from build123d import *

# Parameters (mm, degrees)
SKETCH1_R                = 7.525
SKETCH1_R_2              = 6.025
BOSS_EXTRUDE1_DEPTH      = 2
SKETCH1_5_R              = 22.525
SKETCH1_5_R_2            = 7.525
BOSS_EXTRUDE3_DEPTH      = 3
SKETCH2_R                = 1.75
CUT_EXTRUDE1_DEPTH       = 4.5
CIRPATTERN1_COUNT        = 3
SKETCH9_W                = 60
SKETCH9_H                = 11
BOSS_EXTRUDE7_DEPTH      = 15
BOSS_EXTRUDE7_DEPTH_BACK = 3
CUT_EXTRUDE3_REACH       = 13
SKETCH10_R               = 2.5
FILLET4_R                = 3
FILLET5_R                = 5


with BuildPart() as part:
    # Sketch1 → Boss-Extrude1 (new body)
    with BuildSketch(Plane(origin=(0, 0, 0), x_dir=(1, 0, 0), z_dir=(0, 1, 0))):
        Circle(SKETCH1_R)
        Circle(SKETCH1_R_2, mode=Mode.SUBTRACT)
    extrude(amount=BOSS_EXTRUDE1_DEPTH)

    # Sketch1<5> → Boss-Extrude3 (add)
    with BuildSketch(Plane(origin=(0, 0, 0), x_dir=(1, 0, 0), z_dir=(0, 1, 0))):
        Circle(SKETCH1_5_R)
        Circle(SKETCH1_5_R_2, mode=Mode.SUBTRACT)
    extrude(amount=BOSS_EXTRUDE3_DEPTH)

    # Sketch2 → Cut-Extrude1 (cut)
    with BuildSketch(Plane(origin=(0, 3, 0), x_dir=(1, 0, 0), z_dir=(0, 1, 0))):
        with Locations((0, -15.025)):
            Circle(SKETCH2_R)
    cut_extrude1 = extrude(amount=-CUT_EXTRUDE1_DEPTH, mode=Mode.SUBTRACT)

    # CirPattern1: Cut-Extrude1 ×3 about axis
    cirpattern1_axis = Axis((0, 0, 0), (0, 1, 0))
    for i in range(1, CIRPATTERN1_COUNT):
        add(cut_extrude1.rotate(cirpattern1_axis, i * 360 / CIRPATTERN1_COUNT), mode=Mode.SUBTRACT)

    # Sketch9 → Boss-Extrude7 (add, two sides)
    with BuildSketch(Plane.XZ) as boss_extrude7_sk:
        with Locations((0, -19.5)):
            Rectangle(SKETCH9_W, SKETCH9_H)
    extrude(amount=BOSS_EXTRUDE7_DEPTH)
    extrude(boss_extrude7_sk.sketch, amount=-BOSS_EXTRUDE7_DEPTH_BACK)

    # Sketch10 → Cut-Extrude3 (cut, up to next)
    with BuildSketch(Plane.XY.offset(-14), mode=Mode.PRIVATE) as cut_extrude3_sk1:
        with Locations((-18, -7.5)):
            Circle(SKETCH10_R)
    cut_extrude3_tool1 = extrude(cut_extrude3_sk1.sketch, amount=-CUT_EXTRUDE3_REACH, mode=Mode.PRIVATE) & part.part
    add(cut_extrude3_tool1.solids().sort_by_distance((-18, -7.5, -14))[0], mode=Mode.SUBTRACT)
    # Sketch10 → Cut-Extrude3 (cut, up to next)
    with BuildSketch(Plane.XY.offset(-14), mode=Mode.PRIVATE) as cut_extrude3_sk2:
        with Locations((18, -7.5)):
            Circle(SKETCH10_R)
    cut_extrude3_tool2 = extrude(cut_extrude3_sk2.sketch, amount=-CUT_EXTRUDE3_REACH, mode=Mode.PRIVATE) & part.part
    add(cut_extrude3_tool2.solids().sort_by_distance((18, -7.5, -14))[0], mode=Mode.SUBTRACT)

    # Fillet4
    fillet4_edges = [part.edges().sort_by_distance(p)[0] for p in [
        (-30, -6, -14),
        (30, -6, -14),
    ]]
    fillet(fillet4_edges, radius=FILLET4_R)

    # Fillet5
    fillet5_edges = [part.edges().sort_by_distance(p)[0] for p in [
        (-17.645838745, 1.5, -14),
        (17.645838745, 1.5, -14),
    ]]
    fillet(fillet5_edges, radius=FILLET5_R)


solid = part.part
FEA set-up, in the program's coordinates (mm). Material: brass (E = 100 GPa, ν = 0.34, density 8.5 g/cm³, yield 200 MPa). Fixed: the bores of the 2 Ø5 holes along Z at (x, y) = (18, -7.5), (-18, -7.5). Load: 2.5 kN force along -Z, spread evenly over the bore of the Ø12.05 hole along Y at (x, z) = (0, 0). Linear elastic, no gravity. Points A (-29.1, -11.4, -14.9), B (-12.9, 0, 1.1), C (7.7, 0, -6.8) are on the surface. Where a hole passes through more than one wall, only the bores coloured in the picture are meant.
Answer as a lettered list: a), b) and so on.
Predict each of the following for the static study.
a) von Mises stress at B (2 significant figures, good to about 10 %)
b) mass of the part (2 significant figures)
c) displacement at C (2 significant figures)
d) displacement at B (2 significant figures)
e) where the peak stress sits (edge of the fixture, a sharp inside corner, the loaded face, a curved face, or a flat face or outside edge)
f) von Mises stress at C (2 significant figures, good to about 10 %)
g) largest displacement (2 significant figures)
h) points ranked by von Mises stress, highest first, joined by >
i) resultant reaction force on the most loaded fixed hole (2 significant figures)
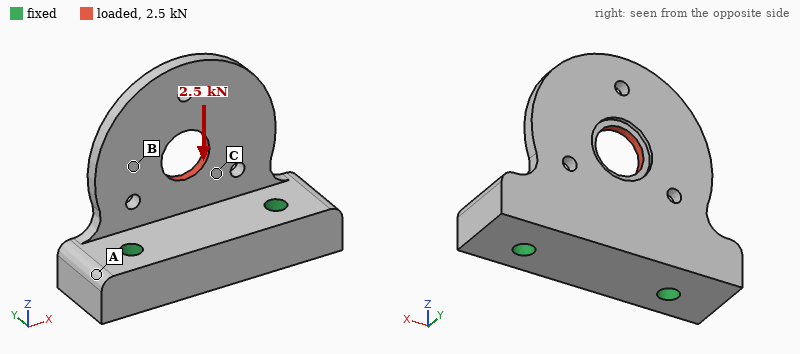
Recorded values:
a) 24 MPa
b) 130 g
c) 7.7 µm
d) 11 µm
e) a curved face
f) 45 MPa
g) 46 µm
h) C > B > A
i) 1.3 kN
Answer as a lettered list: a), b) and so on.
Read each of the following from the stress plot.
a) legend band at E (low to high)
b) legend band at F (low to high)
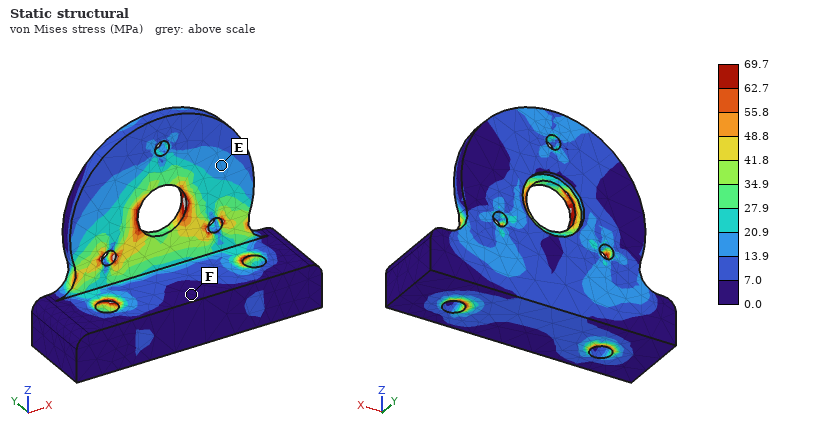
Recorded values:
a) 13.9 to 20.9 MPa
b) 0.0 to 7.0 MPa
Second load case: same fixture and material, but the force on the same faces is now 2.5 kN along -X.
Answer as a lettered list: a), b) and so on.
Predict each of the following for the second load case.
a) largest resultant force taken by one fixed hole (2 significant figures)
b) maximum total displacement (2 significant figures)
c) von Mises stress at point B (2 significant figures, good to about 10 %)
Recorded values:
a) 1.8 kN
b) 32 µm
c) 40 MPa
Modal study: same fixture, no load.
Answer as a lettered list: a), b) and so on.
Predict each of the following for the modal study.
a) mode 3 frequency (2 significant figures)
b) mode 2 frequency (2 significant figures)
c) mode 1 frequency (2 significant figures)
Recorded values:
a) 6700 Hz
b) 3200 Hz
c) 1300 Hz
